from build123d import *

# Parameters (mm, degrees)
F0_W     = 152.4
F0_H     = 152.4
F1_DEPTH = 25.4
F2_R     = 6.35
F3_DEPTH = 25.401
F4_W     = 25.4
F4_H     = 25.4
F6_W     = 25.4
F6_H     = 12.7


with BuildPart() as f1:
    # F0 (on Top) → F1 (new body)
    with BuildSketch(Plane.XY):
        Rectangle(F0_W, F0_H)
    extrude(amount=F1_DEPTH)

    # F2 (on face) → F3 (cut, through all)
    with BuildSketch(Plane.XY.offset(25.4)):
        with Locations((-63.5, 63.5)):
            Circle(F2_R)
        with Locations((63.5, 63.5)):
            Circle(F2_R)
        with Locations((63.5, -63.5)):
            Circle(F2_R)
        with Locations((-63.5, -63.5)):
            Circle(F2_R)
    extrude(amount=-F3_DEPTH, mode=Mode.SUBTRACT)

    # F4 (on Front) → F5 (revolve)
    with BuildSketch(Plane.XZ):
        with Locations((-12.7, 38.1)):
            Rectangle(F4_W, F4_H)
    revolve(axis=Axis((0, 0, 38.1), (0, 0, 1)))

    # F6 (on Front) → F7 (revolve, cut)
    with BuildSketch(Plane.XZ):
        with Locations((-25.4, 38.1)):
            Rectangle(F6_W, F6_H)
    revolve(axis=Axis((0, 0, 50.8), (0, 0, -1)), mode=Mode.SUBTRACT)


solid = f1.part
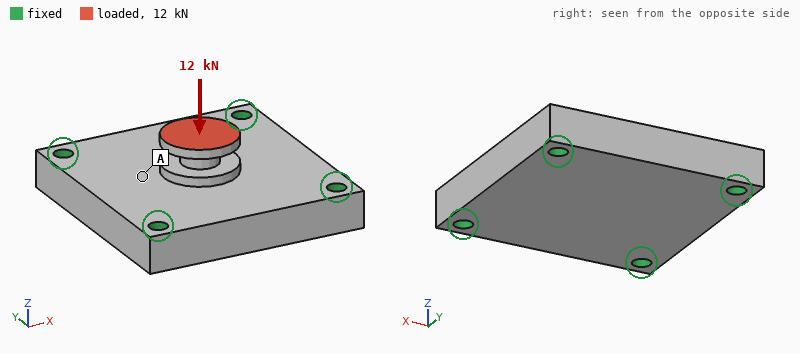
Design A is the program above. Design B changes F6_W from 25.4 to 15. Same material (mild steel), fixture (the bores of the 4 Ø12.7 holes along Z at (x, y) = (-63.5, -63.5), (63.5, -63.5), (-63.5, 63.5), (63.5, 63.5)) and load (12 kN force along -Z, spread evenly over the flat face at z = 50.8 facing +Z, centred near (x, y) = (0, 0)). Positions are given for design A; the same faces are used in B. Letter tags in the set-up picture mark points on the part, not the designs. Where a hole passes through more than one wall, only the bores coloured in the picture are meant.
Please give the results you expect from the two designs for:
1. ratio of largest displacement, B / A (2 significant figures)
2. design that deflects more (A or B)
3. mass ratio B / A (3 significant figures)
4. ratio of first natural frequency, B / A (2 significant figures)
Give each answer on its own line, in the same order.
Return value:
0.56
A
1.01
0.99
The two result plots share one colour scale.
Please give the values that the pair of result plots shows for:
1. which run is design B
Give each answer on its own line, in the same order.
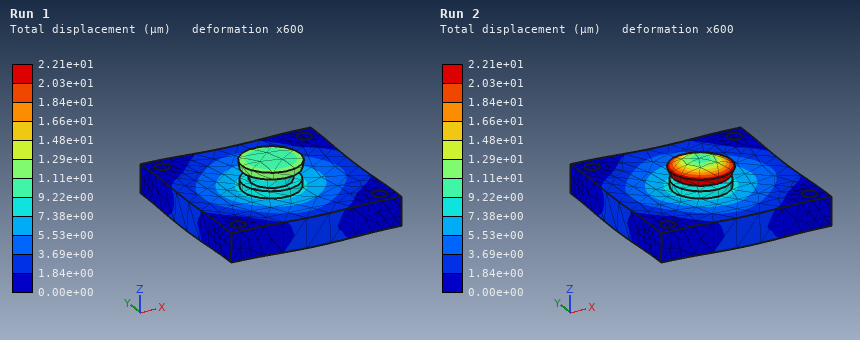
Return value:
Run 1
